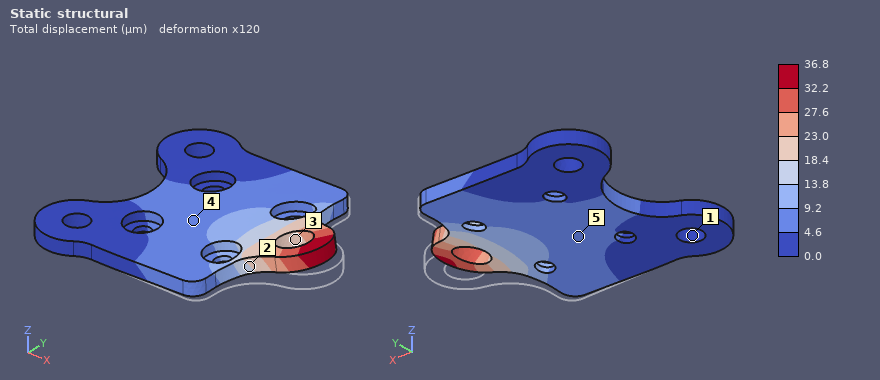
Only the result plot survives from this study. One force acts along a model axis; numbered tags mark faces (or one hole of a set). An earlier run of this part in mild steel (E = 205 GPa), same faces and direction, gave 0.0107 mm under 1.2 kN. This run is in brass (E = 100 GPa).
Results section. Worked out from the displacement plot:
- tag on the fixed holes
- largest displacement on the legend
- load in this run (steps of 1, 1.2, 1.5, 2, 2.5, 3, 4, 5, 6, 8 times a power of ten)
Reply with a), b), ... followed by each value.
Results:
a) 1
b) 36.8 µm
c) 2 kN
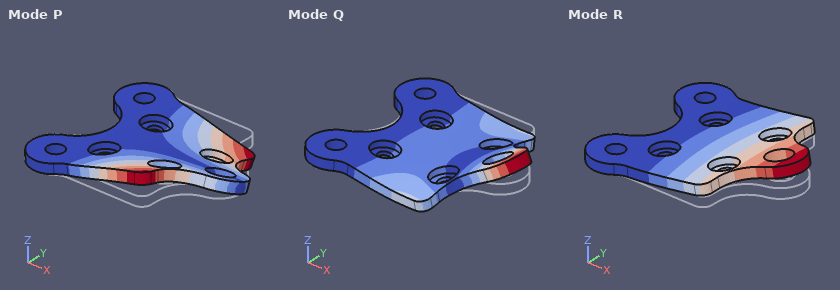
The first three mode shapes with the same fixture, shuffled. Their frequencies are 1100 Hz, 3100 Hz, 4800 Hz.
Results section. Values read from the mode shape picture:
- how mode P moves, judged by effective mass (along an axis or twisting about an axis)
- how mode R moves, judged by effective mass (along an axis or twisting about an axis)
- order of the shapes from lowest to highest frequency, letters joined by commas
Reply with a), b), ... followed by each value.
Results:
a) twisting about X
b) along Z
c) R, P, Q
